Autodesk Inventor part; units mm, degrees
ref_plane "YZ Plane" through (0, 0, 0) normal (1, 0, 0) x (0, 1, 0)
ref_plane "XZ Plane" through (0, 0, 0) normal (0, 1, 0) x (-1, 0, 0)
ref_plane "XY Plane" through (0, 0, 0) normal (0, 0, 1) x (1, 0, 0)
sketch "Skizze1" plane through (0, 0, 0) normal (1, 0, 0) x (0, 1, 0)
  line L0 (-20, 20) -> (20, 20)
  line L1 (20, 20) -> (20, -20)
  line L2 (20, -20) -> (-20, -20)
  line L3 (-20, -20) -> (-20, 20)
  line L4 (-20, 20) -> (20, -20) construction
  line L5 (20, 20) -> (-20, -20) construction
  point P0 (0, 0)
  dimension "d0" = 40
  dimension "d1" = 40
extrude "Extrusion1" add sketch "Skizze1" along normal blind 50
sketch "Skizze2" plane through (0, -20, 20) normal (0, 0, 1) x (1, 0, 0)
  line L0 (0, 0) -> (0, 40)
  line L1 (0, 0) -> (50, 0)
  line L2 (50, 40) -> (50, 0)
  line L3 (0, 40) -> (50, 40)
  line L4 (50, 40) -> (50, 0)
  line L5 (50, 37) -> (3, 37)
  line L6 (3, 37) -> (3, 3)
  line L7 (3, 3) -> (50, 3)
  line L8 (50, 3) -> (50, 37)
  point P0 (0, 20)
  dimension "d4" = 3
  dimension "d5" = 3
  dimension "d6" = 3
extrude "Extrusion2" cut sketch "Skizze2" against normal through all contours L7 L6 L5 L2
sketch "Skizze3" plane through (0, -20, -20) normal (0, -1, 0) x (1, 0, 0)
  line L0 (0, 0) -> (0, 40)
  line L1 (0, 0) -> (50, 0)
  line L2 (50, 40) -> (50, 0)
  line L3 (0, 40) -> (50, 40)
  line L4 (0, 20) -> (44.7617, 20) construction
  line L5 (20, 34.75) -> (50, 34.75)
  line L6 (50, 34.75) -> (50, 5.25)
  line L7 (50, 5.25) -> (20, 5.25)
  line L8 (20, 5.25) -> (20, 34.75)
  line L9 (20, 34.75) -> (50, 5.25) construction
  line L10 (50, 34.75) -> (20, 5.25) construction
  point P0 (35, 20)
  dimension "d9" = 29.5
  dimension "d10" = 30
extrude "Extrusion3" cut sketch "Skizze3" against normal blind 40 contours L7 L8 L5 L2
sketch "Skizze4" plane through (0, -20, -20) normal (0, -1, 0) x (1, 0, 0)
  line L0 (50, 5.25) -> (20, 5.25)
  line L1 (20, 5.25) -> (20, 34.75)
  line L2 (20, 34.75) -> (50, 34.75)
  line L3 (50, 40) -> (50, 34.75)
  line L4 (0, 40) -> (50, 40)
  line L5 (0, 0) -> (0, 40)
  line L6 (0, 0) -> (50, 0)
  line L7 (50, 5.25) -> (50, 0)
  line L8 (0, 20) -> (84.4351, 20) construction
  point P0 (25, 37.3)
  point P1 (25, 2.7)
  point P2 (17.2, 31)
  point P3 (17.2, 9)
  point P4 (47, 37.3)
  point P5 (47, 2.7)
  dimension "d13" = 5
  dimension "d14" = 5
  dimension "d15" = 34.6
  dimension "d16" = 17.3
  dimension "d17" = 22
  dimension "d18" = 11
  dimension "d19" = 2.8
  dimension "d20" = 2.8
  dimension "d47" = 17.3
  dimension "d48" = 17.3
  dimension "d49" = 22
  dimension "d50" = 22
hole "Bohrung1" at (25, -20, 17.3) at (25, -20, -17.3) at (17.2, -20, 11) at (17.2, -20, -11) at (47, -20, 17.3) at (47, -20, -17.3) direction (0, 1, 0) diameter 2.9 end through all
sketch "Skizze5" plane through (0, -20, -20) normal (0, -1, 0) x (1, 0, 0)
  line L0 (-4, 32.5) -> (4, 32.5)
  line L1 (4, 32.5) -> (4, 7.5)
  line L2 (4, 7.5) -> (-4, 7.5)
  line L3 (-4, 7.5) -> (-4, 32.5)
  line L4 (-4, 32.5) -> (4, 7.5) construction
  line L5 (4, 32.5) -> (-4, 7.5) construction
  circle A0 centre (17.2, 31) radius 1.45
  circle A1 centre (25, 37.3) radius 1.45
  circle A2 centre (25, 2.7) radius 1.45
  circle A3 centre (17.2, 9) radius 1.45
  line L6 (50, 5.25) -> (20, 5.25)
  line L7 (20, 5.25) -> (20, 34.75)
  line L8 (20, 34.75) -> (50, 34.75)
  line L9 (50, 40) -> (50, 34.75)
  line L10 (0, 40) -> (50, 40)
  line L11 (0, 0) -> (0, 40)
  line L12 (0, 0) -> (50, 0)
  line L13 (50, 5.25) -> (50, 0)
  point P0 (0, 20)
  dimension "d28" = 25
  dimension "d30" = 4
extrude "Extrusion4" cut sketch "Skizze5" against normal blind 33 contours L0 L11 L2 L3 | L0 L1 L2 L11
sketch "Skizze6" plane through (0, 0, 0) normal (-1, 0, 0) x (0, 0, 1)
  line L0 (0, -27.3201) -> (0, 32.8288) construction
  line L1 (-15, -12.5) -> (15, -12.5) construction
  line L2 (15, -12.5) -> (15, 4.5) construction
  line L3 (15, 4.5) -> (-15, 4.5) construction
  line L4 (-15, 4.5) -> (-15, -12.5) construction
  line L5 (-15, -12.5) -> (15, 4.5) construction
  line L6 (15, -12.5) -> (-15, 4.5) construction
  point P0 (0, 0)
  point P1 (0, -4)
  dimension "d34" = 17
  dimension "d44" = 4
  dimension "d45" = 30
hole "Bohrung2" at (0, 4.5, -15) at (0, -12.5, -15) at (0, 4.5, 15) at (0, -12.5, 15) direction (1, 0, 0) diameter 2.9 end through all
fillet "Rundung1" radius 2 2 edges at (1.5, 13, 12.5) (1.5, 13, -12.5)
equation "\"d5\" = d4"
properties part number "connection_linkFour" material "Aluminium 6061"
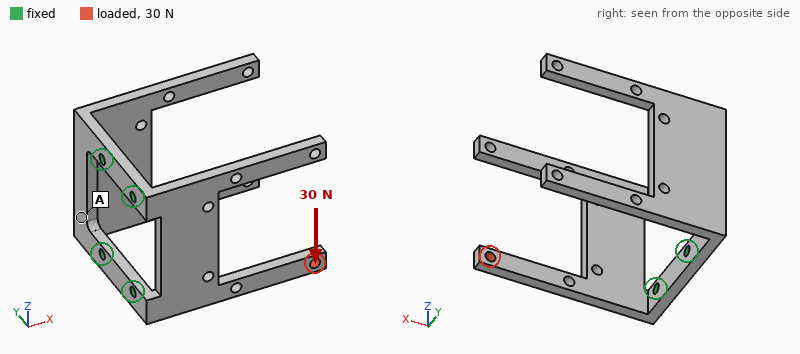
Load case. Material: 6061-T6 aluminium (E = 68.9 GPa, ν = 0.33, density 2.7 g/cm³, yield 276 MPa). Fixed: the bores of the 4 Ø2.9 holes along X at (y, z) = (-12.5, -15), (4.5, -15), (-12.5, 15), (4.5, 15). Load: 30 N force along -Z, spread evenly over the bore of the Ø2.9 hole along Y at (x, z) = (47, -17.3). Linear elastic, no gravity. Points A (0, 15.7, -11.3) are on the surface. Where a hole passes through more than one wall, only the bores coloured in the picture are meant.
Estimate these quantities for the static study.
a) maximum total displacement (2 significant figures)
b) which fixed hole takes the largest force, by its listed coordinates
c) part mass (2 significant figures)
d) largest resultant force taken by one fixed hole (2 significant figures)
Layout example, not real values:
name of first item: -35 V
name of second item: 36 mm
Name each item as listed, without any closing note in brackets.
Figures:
maximum total displacement: 0.15 mm
which fixed hole takes the largest force, by its listed coordinates: (-12.5, 15)
part mass: 21 g
largest resultant force taken by one fixed hole: 53 N
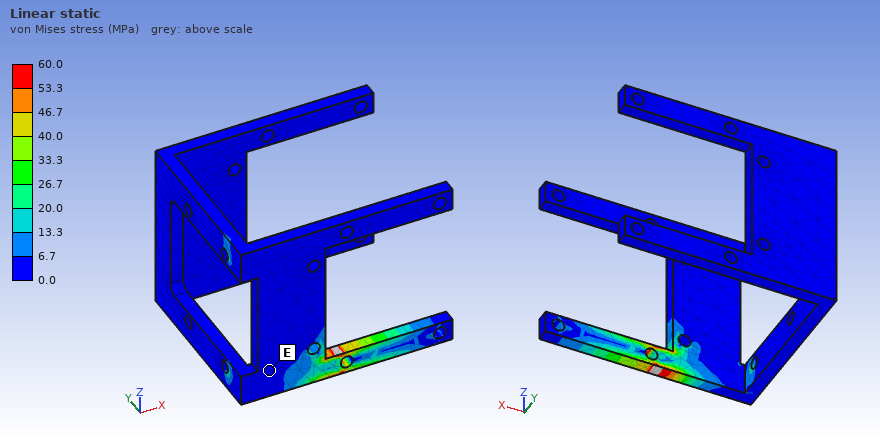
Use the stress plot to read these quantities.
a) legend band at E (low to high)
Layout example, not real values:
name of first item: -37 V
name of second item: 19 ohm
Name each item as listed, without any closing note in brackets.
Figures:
legend band at E: 0.0 to 6.7 MPa
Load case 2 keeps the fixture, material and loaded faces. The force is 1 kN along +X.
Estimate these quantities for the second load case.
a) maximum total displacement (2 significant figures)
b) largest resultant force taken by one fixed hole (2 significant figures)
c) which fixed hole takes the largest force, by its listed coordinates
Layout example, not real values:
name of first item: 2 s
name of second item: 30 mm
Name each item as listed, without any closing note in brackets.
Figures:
maximum total displacement: 0.44 mm
largest resultant force taken by one fixed hole: 1.1 kN
which fixed hole takes the largest force, by its listed coordinates: (-12.5, -15)
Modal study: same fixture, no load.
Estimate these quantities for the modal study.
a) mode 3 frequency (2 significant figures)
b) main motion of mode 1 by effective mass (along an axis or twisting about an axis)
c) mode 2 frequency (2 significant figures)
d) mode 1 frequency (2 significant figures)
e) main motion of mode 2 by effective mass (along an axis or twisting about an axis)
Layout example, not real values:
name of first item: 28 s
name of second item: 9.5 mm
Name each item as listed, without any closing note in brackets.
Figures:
mode 3 frequency: 1500 Hz
main motion of mode 1 by effective mass: along Y
mode 2 frequency: 1100 Hz
mode 1 frequency: 950 Hz
main motion of mode 2 by effective mass: along Y
